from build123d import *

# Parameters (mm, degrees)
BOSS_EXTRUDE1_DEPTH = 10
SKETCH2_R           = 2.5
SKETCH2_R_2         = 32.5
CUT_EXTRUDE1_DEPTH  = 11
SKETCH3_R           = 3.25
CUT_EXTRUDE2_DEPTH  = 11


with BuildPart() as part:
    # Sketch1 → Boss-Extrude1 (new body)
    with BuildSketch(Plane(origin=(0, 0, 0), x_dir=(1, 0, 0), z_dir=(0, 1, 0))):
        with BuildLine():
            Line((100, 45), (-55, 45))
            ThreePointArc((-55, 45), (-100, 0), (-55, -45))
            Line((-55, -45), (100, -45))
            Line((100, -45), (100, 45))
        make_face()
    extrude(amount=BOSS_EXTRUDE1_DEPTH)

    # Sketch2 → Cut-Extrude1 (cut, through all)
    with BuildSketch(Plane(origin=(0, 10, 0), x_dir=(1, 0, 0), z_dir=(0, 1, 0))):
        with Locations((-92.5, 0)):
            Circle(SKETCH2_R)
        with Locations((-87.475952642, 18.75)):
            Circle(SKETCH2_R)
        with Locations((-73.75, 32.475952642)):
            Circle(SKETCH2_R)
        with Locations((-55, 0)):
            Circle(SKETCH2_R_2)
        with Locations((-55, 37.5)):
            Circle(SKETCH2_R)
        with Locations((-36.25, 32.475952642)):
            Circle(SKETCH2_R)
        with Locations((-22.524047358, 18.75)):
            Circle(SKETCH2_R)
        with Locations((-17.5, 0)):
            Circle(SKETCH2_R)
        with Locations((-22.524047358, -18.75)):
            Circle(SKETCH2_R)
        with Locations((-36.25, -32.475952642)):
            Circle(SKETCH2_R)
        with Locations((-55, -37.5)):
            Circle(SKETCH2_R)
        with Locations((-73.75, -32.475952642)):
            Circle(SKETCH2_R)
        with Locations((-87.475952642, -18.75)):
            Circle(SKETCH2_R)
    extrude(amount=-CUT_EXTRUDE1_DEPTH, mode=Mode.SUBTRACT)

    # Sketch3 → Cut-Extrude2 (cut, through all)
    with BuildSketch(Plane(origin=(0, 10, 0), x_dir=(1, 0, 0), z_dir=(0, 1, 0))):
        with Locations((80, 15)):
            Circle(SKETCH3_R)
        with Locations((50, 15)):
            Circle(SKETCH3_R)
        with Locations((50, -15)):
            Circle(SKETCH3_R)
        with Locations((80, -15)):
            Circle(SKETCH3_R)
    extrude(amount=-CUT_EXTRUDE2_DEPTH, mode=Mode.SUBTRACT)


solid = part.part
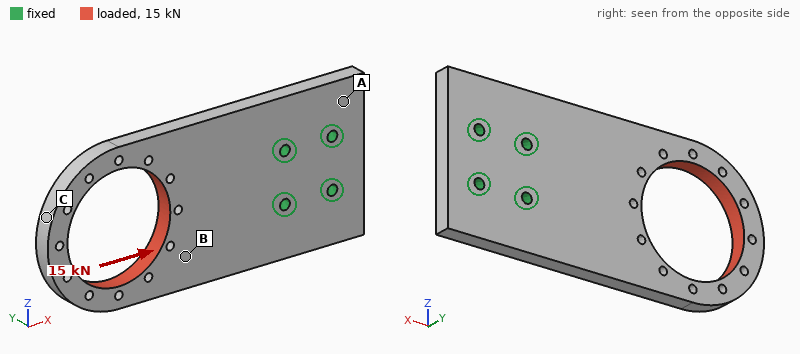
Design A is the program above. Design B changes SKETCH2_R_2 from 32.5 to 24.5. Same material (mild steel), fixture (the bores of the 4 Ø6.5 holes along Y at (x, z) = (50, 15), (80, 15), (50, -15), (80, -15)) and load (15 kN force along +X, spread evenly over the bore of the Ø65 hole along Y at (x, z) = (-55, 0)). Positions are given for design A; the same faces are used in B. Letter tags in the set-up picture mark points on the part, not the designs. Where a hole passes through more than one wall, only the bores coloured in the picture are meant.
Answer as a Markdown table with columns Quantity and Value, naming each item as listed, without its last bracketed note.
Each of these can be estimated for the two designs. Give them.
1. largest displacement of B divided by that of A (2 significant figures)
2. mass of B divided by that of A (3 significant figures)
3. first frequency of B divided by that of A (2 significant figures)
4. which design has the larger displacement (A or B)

| Quantity | Value |
|---|---|
| largest displacement of B divided by that of A | 0.44 |
| mass of B divided by that of A | 1.11 |
| first frequency of B divided by that of A | 0.88 |
| which design has the larger displacement | A |
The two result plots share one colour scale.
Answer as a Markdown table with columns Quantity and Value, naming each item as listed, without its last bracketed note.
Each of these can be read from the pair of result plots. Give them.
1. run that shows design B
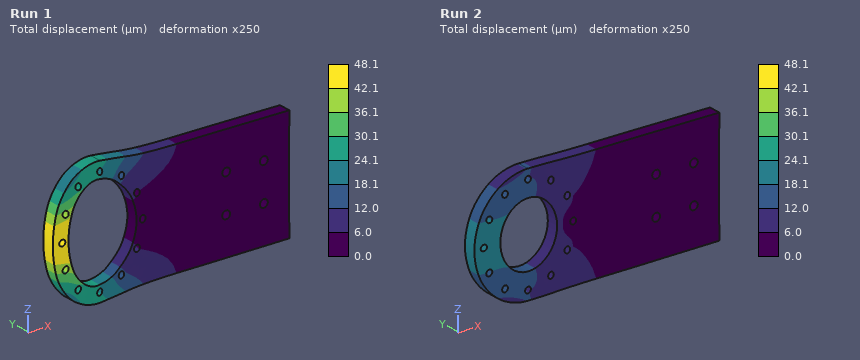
| Quantity | Value |
|---|---|
| run that shows design B | Run 2 |
